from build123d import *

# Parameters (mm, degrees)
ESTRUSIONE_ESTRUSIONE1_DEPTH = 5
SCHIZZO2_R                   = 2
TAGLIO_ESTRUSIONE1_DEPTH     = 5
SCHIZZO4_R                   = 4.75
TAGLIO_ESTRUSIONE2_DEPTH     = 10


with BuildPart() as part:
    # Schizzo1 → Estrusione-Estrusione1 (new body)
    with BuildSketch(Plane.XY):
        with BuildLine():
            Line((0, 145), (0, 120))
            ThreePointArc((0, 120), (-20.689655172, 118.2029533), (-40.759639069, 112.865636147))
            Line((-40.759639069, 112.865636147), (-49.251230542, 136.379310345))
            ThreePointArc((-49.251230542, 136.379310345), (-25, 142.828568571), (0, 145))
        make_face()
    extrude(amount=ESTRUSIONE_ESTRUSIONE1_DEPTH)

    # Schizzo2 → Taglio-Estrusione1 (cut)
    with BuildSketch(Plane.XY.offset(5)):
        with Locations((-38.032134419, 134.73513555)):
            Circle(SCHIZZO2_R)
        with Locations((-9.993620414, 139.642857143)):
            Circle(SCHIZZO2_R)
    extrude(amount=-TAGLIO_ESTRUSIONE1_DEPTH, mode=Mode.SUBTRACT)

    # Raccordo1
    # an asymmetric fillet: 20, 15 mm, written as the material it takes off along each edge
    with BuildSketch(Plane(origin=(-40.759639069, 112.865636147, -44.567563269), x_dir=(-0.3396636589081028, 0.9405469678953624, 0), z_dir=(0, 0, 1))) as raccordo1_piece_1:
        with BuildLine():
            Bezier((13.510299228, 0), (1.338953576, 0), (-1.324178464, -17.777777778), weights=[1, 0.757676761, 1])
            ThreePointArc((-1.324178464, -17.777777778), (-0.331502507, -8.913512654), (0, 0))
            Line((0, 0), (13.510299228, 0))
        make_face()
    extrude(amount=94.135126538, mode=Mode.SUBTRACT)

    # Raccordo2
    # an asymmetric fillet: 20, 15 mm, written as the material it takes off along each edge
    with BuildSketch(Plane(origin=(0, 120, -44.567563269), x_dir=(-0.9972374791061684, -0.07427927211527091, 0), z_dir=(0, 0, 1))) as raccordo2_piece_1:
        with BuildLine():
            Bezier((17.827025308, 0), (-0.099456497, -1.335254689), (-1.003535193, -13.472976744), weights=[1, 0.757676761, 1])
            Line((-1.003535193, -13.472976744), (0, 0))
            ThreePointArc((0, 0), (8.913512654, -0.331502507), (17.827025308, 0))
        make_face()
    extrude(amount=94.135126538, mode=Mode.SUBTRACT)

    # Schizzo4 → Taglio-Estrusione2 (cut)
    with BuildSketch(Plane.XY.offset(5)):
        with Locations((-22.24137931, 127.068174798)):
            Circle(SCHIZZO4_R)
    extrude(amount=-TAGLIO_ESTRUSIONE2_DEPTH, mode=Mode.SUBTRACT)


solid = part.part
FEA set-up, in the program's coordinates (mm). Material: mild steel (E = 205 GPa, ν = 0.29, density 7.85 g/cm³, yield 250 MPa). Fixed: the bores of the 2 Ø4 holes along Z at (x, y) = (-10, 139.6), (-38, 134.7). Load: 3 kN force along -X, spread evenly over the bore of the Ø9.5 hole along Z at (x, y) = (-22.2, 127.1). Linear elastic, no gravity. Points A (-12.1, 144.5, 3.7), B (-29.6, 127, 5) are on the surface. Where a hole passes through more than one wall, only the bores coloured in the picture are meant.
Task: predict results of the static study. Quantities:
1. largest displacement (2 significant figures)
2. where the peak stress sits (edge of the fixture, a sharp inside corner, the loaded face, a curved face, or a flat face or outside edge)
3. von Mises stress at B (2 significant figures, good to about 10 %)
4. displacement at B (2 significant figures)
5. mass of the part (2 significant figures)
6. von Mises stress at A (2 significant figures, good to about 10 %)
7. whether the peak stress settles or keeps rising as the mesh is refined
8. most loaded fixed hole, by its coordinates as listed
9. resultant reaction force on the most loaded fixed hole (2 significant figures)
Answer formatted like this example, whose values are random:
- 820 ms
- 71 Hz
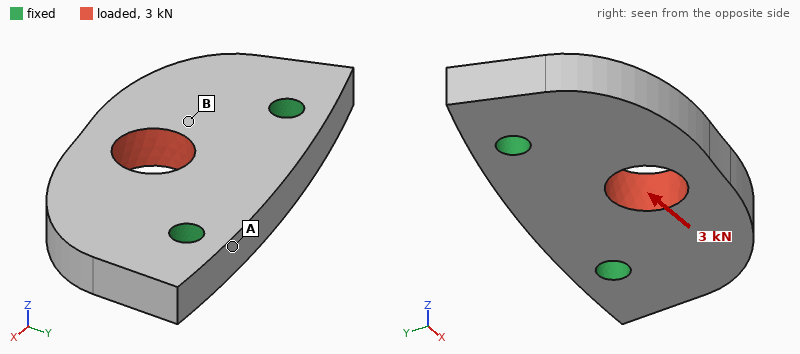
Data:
- 5.2 µm
- edge of the fixture
- 39 MPa
- 2.6 µm
- 37 g
- 14 MPa
- keeps rising
- (-38, 134.7)
- 1.9 kN
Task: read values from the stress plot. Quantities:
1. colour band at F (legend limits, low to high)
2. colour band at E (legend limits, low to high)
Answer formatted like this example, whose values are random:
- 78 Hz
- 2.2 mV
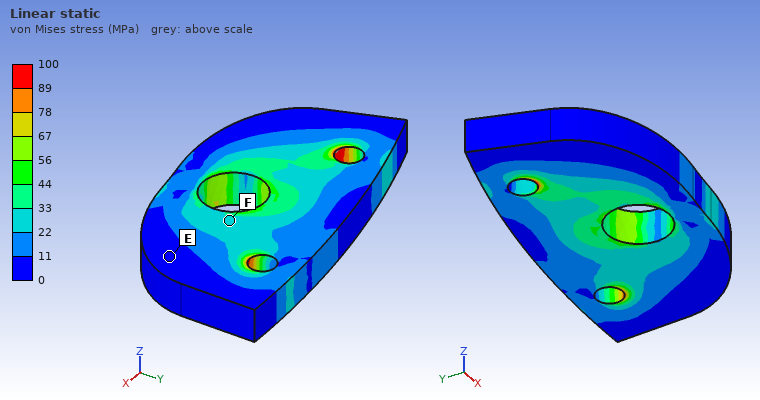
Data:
- 22 to 33 MPa
- 0 to 11 MPa
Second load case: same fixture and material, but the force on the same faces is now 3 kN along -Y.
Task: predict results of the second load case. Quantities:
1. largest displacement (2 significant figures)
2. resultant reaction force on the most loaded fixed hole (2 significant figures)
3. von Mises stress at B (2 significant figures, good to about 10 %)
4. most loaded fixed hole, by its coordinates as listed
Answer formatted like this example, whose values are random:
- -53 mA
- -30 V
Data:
- 4.2 µm
- 1.8 kN
- 28 MPa
- (-10, 139.6)
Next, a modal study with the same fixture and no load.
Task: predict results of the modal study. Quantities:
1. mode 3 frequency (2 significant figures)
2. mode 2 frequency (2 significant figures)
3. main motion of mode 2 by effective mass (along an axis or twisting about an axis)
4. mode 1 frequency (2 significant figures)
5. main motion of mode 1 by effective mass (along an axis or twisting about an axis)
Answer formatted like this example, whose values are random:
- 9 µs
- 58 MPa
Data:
- 26 kHz
- 19 kHz
- twisting about Y
- 11 kHz
- along Z
